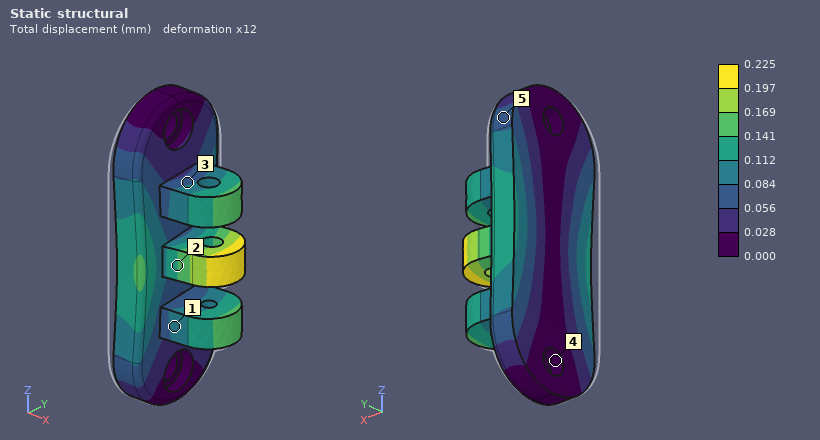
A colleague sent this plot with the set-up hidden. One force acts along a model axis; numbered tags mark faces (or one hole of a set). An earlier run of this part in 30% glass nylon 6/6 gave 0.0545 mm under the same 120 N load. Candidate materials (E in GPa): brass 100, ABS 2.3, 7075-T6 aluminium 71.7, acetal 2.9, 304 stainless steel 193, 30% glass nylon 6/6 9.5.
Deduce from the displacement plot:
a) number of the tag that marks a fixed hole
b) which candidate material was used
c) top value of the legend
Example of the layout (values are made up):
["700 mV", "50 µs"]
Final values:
["4", "ABS", "0.225 mm"]
